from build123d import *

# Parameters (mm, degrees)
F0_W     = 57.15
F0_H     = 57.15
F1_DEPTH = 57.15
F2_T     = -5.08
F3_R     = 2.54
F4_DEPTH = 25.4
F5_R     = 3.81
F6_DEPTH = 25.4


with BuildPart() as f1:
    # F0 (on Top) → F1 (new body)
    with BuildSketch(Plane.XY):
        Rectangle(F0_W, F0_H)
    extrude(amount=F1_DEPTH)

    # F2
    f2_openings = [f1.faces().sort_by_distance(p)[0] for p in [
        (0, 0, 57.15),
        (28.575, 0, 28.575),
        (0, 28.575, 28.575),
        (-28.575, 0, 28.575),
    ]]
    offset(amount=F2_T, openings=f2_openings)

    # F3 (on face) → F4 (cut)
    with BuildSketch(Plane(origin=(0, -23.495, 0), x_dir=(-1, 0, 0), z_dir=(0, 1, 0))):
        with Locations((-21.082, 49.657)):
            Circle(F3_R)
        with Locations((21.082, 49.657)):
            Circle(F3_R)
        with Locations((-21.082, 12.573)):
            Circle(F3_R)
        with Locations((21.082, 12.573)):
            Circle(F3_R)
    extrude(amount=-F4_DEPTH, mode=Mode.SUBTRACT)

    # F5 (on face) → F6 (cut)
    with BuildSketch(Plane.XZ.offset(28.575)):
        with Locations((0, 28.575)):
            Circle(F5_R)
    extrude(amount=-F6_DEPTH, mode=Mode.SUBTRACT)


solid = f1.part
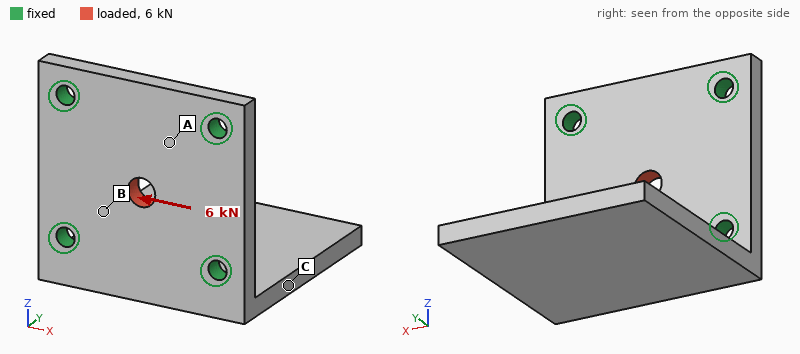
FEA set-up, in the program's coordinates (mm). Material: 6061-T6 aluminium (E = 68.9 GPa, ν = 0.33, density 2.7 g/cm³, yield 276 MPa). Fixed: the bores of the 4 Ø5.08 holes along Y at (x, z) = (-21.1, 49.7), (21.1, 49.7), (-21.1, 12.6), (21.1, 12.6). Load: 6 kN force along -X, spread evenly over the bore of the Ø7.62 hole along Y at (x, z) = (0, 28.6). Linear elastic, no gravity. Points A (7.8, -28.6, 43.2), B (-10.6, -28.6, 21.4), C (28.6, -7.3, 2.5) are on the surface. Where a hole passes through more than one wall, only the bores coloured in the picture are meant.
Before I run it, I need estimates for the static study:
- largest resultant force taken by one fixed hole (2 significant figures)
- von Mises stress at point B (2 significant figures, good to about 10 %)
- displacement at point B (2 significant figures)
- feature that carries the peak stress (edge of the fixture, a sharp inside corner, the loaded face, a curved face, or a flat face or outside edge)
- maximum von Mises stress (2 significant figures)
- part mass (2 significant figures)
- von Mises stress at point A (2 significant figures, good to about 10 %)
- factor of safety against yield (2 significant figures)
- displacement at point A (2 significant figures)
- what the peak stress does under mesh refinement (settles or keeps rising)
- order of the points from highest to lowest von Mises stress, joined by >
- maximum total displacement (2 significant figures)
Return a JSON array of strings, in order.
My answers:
["1.8 kN", "28 MPa", "5.7 µm", "the loaded face", "86 MPa", "84 g", "17 MPa", "3.2", "3.7 µm", "settles", "B > A > C", "12 µm"]
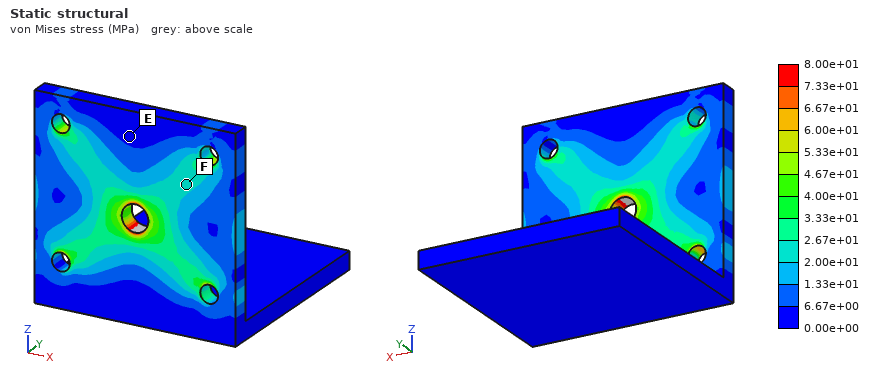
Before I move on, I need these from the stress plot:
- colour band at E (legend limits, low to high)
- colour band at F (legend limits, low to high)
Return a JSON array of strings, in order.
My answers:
["0.00e+00 to 6.67e+00 MPa", "2.00e+01 to 2.67e+01 MPa"]
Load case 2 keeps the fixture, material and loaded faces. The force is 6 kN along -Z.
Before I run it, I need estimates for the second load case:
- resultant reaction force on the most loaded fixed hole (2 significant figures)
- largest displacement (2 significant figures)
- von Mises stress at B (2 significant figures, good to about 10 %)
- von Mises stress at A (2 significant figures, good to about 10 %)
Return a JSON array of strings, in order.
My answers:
["1.7 kN", "13 µm", "24 MPa", "21 MPa"]
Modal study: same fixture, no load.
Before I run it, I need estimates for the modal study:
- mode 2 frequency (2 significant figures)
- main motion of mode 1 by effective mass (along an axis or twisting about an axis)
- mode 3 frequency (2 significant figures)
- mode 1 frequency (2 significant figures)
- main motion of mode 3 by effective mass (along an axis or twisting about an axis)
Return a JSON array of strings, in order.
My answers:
["2900 Hz", "along Z", "4900 Hz", "1100 Hz", "along X"]
